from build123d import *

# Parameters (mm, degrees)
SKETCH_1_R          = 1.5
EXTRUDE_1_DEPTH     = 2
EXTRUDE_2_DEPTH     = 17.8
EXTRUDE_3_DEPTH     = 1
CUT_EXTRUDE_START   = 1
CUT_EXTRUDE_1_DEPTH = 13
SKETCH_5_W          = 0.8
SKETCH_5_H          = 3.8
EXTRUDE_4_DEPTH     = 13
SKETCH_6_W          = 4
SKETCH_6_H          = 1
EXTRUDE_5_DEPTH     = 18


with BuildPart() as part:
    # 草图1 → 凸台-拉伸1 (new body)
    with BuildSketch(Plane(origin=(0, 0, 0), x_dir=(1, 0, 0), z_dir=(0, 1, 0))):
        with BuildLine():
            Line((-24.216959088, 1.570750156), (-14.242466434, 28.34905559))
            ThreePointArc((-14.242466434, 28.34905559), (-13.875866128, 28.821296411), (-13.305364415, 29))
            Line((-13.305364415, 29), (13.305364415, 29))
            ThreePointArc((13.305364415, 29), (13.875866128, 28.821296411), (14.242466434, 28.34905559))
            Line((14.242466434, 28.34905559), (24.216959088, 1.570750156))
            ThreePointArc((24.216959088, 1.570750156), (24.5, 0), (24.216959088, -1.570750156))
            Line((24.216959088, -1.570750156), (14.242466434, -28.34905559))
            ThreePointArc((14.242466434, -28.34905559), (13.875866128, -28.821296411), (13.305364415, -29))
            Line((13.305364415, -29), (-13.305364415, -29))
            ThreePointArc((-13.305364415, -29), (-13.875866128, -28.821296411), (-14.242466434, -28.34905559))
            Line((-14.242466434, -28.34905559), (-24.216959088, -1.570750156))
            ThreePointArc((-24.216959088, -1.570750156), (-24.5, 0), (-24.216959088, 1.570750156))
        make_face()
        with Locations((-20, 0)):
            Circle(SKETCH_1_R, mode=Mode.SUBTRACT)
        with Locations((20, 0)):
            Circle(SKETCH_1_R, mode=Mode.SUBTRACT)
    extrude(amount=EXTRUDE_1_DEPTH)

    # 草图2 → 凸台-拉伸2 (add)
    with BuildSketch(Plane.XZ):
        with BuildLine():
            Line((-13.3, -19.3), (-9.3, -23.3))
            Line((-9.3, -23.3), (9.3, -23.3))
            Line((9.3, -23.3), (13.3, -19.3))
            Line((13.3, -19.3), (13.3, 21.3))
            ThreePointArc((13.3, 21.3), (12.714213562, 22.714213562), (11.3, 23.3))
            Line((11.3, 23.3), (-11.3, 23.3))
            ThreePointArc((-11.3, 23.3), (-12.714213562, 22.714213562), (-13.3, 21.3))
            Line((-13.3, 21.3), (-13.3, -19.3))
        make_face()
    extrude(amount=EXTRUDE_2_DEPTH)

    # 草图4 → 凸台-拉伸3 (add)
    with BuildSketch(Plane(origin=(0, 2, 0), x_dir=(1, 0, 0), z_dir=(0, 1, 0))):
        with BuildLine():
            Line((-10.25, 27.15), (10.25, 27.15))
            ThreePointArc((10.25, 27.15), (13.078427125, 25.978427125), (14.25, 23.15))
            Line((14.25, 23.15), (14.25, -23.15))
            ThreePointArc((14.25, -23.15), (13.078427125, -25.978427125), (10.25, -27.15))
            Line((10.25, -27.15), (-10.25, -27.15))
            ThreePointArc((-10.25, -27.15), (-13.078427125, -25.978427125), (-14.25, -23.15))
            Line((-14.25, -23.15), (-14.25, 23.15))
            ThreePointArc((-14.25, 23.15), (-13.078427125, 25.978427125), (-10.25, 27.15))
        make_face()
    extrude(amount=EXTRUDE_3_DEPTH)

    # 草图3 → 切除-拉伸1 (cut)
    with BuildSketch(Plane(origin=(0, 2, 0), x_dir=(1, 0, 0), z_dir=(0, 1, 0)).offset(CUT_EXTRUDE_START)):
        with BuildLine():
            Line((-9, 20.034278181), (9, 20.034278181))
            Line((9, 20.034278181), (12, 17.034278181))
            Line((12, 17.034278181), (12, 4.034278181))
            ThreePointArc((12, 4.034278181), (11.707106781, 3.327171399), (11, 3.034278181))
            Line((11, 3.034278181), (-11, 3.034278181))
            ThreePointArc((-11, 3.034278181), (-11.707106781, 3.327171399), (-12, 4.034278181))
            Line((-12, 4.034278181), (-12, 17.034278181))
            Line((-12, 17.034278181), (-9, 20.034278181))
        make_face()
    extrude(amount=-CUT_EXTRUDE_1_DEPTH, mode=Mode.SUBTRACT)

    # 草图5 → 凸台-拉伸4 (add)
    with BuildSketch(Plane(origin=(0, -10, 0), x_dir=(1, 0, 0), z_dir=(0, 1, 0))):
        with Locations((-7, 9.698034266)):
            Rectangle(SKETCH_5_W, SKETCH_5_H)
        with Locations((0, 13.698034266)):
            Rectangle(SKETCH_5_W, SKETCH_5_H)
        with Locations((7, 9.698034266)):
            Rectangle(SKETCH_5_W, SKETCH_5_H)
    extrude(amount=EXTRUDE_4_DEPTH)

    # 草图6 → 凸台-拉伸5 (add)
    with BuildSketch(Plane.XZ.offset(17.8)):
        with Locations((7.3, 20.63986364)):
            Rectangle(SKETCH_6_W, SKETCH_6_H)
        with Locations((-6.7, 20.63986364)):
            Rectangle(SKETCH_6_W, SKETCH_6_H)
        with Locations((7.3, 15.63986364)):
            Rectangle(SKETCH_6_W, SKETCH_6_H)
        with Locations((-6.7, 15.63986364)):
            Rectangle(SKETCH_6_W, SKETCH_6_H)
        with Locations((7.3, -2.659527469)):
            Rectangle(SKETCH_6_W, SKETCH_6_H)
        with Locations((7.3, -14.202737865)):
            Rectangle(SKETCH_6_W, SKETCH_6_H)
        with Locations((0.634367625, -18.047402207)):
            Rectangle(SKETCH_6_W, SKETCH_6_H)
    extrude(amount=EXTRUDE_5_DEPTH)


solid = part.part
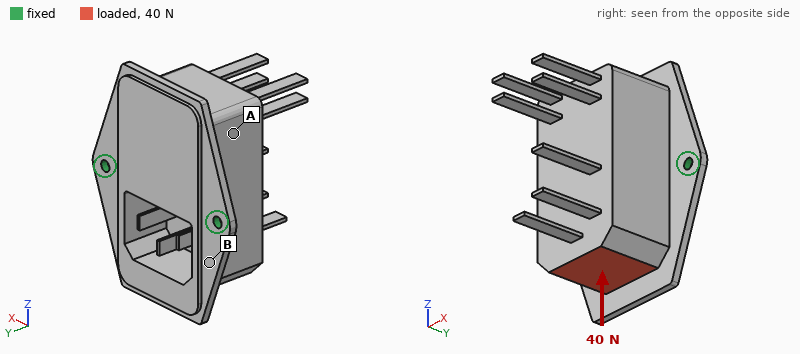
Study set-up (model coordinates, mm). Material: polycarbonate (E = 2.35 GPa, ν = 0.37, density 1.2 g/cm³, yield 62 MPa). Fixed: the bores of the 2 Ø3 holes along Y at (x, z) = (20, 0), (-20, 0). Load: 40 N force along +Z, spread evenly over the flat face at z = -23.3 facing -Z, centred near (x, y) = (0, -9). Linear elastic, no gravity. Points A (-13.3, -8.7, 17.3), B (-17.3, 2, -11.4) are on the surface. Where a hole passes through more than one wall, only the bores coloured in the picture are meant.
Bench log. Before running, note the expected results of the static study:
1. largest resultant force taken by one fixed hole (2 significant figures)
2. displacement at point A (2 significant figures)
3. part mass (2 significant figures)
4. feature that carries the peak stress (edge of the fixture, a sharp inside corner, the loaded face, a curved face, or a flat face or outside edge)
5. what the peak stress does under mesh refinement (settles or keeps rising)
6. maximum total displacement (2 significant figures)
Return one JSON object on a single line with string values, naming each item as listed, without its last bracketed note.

{"largest resultant force taken by one fixed hole": "20 N", "displacement at point A": "0.41 mm", "part mass": "28 g", "feature that carries the peak stress": "edge of the fixture", "what the peak stress does under mesh refinement": "keeps rising", "maximum total displacement": "0.88 mm"}
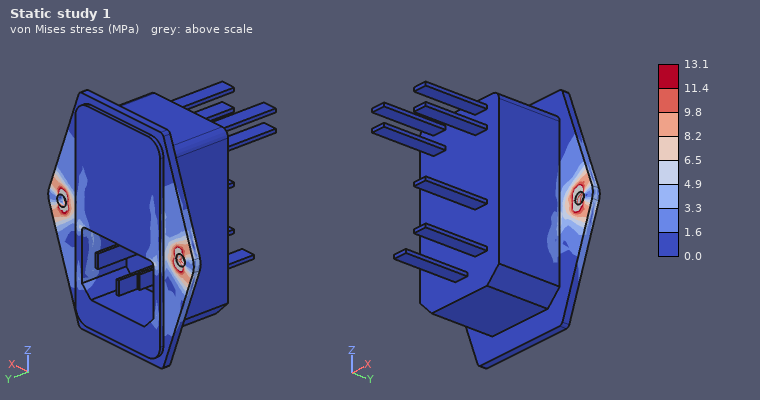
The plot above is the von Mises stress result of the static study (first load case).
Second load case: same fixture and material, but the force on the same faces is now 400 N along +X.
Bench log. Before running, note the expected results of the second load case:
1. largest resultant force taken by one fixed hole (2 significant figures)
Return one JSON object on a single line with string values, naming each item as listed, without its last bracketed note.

{"largest resultant force taken by one fixed hole": "320 N"}
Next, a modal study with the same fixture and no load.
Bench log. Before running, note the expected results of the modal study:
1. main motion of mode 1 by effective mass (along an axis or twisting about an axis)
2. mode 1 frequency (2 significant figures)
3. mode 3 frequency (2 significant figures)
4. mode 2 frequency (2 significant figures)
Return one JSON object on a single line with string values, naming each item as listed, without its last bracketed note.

{"main motion of mode 1 by effective mass": "along Z", "mode 1 frequency": "230 Hz", "mode 3 frequency": "690 Hz", "mode 2 frequency": "690 Hz"}
